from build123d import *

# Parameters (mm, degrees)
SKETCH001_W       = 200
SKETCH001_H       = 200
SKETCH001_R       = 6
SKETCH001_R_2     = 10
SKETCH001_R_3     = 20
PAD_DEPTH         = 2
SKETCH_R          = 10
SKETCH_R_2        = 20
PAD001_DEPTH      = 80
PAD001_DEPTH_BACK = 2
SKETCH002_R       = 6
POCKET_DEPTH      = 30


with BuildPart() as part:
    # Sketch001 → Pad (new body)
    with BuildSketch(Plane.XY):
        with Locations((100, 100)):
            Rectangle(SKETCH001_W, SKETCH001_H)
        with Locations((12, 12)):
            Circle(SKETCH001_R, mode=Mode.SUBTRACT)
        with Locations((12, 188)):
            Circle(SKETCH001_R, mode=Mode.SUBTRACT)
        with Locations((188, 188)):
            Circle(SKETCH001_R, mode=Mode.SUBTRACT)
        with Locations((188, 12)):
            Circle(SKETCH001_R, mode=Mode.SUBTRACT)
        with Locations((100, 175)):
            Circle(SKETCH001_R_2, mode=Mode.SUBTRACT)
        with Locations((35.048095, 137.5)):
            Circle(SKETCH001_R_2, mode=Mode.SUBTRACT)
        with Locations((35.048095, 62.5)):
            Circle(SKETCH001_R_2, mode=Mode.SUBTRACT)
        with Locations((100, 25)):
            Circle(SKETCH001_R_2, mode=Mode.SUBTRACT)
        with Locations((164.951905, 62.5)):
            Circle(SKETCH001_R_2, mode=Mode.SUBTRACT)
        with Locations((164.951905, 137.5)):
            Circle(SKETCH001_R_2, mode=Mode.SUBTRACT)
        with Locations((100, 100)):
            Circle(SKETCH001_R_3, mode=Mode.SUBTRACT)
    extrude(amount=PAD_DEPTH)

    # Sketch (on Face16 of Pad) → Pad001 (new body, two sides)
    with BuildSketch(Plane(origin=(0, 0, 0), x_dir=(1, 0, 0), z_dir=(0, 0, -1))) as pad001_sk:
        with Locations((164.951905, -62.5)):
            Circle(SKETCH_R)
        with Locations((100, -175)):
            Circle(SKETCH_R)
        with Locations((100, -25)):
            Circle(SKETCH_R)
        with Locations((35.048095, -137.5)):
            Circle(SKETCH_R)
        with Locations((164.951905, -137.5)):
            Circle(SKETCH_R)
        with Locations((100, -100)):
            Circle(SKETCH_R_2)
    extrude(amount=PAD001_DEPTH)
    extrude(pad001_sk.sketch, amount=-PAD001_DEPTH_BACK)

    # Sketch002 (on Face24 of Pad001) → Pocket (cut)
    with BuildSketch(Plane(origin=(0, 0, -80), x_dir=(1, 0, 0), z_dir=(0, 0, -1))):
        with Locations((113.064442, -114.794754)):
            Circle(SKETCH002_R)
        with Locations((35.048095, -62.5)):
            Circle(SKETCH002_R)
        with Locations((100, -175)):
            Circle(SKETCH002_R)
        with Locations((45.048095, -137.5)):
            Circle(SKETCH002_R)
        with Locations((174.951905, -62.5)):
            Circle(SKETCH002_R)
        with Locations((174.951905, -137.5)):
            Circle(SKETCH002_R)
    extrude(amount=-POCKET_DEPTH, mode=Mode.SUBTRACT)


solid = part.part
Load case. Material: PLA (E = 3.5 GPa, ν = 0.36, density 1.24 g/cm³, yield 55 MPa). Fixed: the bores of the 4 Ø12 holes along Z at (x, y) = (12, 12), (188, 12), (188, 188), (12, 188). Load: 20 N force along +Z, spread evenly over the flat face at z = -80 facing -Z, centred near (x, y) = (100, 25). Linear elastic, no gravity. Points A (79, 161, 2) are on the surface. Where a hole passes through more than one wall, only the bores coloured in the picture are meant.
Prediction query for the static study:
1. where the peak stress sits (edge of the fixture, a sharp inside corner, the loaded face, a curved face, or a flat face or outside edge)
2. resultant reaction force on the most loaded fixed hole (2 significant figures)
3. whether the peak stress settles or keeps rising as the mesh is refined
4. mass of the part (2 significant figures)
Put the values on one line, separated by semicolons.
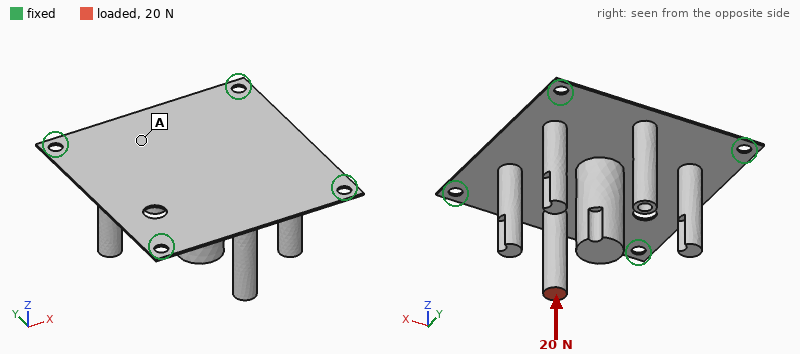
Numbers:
edge of the fixture; 10 N; keeps rising; 370 g
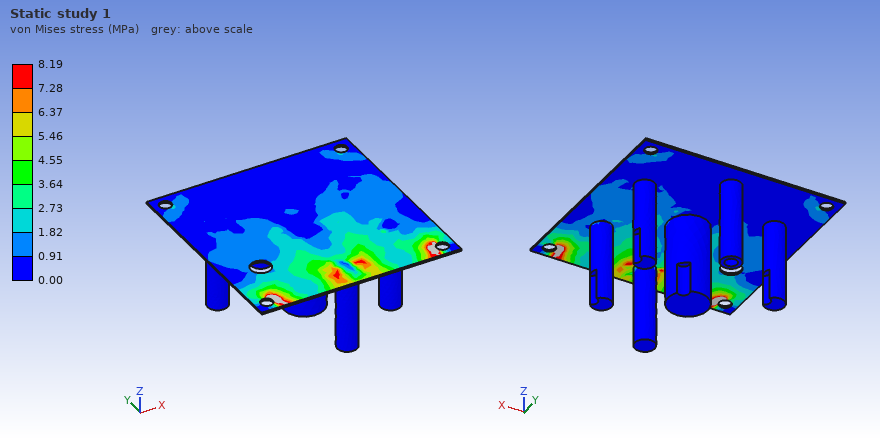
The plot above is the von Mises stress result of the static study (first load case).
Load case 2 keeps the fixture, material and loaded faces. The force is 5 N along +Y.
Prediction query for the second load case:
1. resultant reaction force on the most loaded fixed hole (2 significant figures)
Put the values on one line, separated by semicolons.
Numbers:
2.2 N
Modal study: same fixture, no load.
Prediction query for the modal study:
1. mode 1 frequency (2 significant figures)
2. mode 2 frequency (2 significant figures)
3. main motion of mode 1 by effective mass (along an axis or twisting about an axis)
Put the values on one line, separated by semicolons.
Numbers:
32 Hz; 46 Hz; along Z
